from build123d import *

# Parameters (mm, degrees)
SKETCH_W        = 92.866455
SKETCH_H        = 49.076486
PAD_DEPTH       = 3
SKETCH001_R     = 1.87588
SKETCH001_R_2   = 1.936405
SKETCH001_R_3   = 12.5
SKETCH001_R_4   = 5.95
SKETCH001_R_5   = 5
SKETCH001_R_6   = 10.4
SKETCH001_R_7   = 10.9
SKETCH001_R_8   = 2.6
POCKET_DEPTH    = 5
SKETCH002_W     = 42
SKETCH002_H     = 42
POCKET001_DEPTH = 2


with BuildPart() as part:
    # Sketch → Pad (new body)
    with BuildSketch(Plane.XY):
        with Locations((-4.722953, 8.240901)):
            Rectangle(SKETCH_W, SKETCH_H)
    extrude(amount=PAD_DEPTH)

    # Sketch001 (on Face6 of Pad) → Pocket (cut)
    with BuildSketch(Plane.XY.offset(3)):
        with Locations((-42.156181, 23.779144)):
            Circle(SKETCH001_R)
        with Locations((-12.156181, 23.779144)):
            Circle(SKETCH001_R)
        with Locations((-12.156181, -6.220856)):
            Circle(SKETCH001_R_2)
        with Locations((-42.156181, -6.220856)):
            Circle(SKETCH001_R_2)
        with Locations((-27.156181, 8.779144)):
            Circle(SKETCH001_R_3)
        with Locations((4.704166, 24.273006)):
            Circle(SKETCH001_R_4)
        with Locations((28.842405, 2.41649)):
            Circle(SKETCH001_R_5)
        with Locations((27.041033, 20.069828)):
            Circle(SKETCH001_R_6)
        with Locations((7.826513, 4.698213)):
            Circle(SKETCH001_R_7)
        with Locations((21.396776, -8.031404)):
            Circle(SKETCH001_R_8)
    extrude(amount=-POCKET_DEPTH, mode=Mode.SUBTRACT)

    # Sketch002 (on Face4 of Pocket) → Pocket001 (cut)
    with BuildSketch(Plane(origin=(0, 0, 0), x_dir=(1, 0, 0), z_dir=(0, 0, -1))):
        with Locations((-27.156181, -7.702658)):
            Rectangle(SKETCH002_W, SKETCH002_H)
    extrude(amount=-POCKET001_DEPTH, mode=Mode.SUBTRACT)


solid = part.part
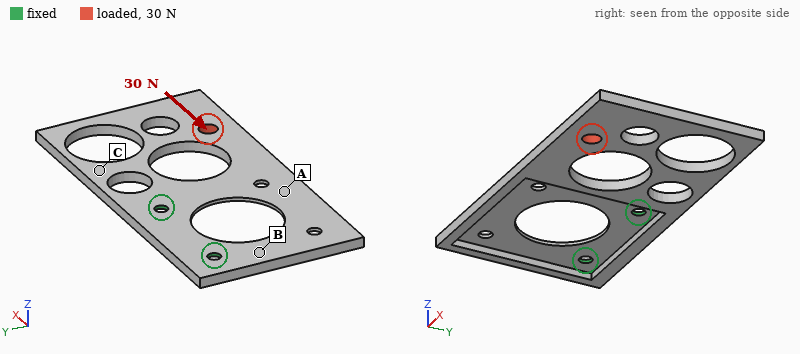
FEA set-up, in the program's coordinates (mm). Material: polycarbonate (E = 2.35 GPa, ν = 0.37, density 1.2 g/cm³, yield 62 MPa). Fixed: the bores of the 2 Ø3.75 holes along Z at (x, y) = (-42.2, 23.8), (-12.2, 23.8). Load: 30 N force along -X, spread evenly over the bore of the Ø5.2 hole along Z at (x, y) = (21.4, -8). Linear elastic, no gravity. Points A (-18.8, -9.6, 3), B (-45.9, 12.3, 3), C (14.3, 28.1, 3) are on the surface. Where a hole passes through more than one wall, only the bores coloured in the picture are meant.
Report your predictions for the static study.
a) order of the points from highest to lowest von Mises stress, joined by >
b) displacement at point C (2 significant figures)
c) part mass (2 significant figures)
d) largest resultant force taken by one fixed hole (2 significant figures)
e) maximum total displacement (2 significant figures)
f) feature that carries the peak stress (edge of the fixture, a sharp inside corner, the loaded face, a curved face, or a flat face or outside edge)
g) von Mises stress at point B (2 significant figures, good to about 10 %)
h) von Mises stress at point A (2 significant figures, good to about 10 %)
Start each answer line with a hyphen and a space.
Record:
- B > A > C
- 0.28 mm
- 8.2 g
- 32 N
- 1.00 mm
- edge of the fixture
- 3.0 MPa
- 1.6 MPa
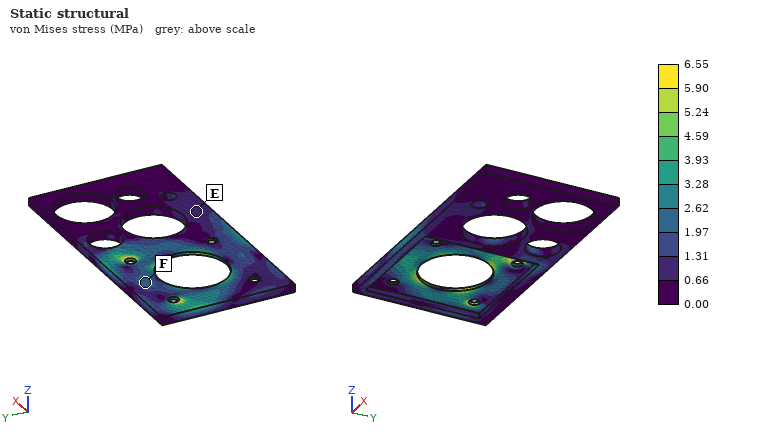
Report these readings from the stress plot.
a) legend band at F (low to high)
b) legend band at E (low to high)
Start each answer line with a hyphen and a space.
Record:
- 1.97 to 2.62 MPa
- 0.66 to 1.31 MPa
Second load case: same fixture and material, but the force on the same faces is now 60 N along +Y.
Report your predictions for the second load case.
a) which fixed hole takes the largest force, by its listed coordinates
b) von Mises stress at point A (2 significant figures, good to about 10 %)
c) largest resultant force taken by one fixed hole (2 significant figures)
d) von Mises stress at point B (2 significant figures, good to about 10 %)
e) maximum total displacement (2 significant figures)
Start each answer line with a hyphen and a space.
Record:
- (-12.2, 23.8)
- 3.3 MPa
- 110 N
- 6.3 MPa
- 1.2 mm
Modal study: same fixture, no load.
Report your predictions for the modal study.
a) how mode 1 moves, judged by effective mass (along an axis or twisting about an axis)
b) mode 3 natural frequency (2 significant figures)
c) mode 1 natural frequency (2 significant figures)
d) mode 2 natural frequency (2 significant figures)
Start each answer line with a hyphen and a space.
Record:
- along Z
- 350 Hz
- 86 Hz
- 180 Hz
